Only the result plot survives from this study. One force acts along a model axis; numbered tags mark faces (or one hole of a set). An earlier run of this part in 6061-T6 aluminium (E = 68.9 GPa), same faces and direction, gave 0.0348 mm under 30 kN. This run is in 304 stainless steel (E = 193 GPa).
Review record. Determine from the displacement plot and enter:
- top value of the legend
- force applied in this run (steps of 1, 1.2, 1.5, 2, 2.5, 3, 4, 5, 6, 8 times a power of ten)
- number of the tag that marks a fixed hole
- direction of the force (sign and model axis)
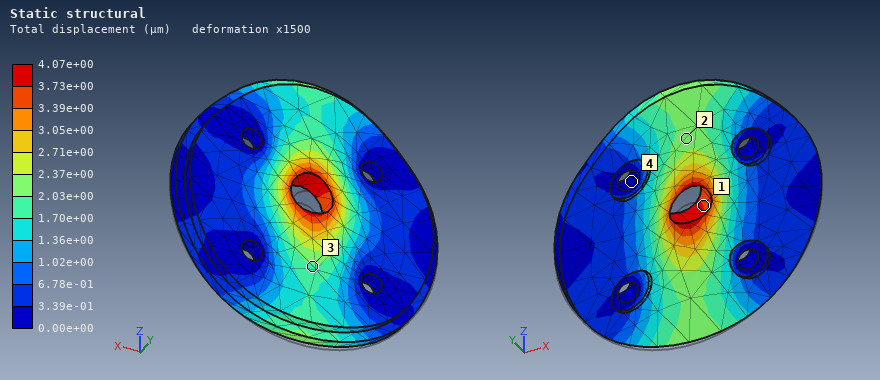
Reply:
4.07e+00 µm
10 kN
4
+Z
